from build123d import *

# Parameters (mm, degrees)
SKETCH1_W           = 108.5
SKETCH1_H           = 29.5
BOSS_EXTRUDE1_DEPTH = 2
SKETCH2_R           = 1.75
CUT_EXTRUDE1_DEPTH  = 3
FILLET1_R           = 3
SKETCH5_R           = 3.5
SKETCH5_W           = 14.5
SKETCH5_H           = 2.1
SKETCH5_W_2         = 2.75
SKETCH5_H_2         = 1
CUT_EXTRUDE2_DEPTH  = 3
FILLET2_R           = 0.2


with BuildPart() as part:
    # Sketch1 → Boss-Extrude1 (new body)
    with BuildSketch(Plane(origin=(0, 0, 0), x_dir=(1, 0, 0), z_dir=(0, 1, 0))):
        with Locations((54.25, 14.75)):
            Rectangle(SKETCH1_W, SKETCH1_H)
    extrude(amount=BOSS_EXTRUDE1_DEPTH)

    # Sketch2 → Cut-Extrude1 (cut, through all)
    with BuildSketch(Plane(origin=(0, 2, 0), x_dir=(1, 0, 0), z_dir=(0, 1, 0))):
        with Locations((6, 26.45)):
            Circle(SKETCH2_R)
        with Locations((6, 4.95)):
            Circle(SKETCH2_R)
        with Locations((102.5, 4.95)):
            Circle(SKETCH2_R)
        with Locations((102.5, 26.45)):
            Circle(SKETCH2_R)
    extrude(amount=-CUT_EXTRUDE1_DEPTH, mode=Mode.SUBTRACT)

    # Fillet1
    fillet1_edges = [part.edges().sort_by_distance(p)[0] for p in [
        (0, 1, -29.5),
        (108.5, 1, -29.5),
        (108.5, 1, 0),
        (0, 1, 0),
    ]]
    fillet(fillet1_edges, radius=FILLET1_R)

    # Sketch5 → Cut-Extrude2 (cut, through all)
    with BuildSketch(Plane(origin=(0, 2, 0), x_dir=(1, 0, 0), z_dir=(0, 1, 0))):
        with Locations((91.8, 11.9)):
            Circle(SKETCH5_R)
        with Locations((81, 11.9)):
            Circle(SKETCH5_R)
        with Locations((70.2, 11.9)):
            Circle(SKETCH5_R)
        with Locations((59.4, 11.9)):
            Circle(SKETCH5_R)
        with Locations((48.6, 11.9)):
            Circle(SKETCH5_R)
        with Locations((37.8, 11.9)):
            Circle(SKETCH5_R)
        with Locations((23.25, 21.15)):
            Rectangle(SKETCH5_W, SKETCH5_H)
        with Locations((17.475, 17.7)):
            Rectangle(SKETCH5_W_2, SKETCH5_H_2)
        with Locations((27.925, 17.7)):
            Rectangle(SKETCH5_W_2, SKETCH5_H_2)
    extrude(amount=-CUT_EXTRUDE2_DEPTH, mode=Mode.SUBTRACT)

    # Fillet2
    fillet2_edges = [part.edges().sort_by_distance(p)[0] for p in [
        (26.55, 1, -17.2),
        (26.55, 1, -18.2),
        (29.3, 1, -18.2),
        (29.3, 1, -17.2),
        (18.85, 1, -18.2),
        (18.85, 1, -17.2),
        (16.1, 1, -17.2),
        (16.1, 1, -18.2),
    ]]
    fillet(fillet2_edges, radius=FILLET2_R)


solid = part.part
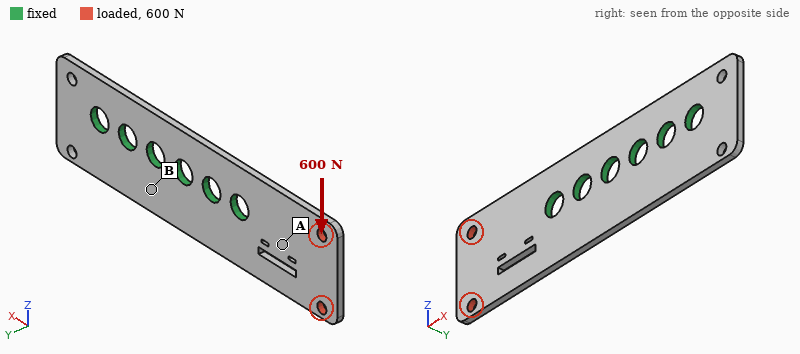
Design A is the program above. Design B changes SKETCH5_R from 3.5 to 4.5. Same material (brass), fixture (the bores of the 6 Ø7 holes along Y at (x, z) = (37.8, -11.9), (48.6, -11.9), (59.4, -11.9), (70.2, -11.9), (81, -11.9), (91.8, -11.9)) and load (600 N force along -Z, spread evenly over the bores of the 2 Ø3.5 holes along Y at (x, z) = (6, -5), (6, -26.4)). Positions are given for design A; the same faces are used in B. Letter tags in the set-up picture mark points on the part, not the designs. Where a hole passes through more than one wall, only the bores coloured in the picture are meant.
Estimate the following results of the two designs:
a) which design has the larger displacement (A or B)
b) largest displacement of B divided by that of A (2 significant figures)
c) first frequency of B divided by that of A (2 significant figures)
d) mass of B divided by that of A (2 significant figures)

A
0.90
1.1
0.95
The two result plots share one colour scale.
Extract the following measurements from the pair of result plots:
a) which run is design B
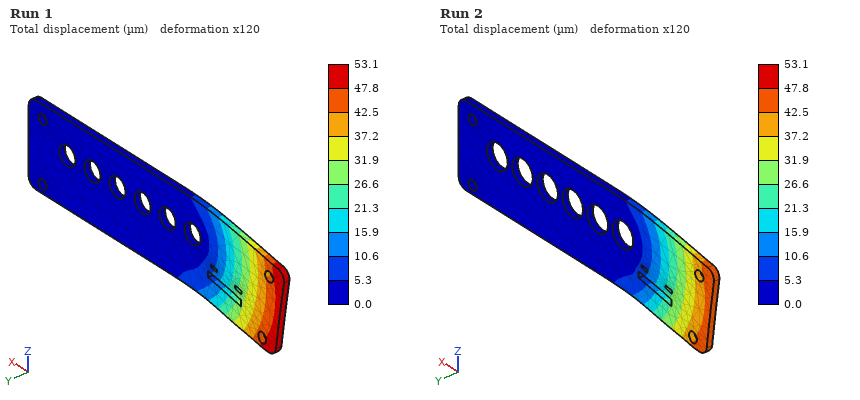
Run 2
